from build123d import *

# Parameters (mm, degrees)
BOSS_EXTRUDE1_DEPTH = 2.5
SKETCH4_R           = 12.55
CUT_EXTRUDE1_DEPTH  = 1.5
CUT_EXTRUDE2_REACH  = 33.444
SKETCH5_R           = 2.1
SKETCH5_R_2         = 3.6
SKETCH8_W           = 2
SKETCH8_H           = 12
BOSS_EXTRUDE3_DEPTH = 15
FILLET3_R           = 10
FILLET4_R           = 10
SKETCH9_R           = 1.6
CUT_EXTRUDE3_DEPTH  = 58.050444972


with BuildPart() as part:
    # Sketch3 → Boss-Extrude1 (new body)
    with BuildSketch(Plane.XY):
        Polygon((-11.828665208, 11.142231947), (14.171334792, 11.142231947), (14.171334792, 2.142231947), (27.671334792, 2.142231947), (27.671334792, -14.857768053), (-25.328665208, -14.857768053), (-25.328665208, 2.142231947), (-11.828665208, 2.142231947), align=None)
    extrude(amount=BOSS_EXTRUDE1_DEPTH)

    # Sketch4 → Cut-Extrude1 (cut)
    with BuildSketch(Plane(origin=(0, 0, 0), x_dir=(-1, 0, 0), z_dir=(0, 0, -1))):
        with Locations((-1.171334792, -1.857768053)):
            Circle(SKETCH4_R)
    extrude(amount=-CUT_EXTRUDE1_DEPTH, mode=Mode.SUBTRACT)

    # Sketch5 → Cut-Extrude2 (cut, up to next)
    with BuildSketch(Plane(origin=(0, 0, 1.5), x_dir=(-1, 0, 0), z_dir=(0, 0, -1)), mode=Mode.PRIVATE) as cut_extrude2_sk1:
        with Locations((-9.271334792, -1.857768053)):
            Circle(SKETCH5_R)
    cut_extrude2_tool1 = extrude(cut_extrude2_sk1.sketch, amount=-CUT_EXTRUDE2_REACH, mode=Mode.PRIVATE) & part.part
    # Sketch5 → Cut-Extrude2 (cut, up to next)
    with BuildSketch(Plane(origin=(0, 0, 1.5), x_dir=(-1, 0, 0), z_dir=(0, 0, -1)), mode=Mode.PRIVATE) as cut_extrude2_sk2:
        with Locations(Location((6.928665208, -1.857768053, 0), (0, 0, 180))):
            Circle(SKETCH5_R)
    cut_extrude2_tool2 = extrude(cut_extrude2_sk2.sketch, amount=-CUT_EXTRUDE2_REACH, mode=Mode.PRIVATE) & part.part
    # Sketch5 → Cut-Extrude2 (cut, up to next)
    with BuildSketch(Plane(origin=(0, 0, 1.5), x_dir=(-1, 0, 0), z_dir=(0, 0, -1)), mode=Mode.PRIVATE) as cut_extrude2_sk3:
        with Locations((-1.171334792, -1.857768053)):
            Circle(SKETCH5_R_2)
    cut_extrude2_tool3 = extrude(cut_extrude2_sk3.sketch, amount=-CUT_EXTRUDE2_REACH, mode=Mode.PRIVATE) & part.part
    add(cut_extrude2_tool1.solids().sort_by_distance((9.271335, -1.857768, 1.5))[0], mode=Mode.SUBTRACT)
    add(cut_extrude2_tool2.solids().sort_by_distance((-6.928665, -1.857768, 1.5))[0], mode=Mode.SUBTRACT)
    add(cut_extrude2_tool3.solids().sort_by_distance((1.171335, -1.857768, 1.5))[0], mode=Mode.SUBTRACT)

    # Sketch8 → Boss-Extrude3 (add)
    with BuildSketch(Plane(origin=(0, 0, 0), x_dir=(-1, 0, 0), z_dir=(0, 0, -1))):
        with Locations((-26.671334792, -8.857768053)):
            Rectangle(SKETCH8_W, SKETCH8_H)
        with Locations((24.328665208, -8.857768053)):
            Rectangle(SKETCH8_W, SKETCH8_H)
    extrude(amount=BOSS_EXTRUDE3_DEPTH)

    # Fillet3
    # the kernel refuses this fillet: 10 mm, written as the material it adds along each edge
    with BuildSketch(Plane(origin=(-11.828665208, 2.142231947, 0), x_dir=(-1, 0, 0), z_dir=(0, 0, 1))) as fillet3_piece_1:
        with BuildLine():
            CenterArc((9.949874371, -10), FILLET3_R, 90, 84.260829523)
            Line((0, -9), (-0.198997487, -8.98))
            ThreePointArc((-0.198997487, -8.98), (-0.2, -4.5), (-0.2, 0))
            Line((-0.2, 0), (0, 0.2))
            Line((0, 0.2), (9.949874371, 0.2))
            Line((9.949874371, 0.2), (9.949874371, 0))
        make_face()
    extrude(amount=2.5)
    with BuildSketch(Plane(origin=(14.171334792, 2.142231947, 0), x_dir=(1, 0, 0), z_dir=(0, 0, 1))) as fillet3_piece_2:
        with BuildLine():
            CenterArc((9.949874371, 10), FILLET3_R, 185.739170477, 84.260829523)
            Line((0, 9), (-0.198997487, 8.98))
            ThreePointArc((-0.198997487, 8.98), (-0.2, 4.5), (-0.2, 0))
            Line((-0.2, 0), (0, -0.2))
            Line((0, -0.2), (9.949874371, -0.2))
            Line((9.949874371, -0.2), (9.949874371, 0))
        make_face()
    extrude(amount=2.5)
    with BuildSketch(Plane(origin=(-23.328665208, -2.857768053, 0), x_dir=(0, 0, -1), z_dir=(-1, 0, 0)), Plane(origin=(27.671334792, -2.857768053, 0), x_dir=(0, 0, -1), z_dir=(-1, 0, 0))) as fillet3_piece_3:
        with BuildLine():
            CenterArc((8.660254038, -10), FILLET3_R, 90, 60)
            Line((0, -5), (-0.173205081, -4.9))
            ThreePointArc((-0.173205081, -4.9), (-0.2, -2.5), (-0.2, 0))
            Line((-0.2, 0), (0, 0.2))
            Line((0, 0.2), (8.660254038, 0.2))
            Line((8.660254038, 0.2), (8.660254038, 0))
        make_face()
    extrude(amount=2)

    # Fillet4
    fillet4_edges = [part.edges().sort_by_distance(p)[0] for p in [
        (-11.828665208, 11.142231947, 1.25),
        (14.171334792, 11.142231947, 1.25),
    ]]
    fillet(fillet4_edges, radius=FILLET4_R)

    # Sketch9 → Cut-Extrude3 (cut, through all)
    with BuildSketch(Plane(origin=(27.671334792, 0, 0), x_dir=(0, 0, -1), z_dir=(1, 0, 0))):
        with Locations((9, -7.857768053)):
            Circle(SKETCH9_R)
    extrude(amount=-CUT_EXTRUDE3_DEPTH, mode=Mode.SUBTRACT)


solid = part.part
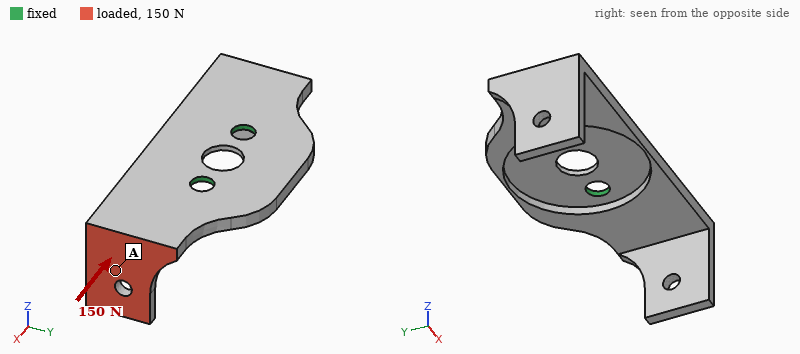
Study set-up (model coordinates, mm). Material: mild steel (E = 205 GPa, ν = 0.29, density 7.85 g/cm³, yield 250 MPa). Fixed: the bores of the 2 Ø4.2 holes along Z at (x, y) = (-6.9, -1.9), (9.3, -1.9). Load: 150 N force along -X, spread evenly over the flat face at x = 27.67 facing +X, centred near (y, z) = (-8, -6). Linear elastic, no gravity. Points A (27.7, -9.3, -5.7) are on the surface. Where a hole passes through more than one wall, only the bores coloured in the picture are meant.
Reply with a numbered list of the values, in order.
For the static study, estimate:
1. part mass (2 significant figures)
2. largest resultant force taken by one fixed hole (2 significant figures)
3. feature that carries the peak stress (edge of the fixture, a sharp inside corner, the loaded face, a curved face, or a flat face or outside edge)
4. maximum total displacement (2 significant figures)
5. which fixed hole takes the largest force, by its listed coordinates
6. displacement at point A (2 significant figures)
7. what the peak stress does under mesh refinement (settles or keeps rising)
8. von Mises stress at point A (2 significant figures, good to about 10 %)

1. 22 g
2. 120 N
3. edge of the fixture
4. 0.18 mm
5. (-6.9, -1.9)
6. 0.11 mm
7. keeps rising
8. 34 MPa
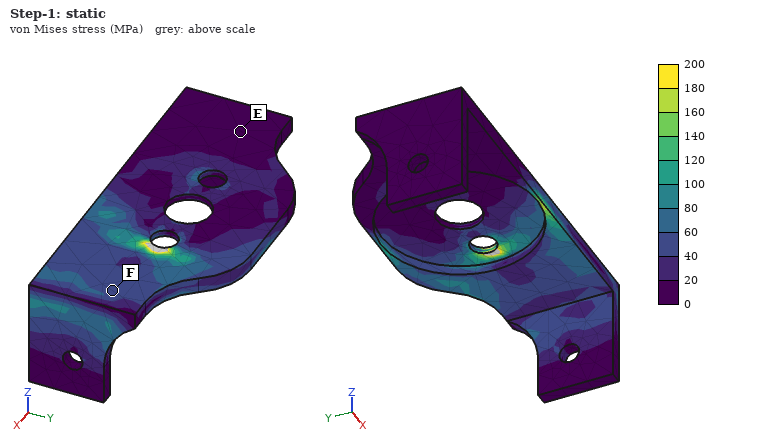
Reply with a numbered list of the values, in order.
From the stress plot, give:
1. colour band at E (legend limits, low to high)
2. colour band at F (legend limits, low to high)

1. 0 to 20 MPa
2. 40 to 60 MPa
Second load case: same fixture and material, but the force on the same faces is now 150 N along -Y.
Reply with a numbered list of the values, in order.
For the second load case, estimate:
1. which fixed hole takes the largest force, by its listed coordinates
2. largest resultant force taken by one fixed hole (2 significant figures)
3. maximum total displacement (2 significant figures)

1. (9.3, -1.9)
2. 260 N
3. 0.12 mm
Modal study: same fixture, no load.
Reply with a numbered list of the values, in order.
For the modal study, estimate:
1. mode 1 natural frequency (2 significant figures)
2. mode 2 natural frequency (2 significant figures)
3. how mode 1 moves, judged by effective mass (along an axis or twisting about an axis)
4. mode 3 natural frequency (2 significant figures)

1. 1700 Hz
2. 1800 Hz
3. along Z
4. 3100 Hz
